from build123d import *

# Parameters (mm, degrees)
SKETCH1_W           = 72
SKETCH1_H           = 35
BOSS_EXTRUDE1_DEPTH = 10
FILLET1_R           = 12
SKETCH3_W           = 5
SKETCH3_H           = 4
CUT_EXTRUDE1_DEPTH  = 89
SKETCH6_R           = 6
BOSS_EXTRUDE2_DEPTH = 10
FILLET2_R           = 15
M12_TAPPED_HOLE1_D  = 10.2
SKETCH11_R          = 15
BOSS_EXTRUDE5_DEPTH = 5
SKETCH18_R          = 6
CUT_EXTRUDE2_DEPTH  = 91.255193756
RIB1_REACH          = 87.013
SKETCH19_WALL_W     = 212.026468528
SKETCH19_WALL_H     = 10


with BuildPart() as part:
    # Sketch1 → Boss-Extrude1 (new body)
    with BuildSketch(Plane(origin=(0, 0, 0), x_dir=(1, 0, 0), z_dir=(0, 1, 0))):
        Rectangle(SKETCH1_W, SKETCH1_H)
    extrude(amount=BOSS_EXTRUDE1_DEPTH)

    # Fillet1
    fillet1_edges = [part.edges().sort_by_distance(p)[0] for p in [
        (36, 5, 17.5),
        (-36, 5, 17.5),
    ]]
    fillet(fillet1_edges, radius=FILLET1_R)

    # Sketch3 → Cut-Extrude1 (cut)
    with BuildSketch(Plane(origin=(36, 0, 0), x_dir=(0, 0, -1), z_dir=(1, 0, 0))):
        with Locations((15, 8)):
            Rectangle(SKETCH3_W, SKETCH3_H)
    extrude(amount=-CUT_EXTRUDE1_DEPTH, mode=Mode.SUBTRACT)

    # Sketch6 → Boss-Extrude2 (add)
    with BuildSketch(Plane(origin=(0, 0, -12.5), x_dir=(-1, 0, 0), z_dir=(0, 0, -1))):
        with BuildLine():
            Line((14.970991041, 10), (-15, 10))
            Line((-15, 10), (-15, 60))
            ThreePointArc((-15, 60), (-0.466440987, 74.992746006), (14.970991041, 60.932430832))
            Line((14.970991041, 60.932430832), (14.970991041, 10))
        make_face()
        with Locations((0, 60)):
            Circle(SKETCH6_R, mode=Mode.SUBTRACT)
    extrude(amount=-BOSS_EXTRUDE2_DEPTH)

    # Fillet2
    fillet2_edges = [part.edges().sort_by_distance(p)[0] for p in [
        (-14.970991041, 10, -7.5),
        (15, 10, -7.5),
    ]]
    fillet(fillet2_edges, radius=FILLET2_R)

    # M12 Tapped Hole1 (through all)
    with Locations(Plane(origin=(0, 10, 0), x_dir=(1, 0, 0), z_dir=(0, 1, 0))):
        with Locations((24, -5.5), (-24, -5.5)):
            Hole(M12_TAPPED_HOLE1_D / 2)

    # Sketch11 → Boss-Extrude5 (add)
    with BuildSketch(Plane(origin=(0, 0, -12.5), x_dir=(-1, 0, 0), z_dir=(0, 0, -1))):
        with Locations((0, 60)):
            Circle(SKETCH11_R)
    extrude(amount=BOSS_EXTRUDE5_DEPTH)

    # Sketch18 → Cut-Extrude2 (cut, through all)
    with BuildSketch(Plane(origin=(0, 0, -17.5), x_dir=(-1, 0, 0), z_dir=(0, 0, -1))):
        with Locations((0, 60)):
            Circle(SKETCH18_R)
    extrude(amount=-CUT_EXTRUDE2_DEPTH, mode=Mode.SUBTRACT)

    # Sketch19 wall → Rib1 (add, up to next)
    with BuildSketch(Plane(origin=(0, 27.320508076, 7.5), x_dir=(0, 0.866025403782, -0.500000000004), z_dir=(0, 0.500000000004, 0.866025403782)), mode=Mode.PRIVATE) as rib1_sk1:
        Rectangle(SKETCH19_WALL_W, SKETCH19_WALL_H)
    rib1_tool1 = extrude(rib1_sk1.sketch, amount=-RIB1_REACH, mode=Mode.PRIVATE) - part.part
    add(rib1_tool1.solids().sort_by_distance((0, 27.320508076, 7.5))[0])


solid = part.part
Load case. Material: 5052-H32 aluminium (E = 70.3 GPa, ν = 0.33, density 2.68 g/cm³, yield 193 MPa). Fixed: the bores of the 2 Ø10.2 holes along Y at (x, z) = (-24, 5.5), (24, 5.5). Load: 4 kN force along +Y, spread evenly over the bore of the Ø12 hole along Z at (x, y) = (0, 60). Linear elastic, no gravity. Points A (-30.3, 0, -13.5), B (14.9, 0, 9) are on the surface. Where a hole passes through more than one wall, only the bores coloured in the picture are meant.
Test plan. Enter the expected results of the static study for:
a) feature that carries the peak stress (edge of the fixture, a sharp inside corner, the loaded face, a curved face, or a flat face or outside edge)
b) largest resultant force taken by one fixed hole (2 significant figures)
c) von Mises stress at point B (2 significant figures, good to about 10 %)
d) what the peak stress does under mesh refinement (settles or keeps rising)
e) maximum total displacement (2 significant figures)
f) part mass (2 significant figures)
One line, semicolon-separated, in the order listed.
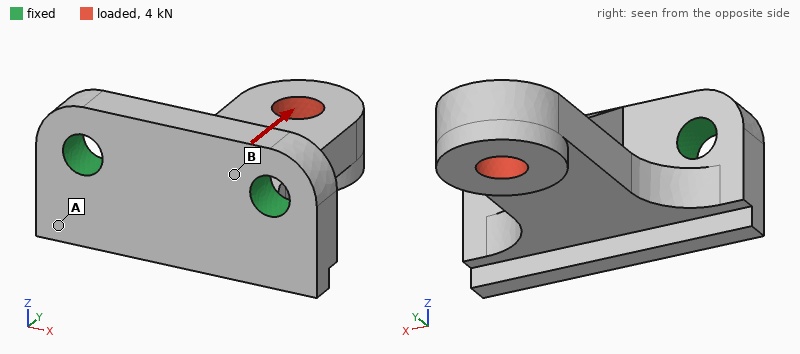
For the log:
edge of the fixture; 2.1 kN; 21 MPa; keeps rising; 0.14 mm; 120 g
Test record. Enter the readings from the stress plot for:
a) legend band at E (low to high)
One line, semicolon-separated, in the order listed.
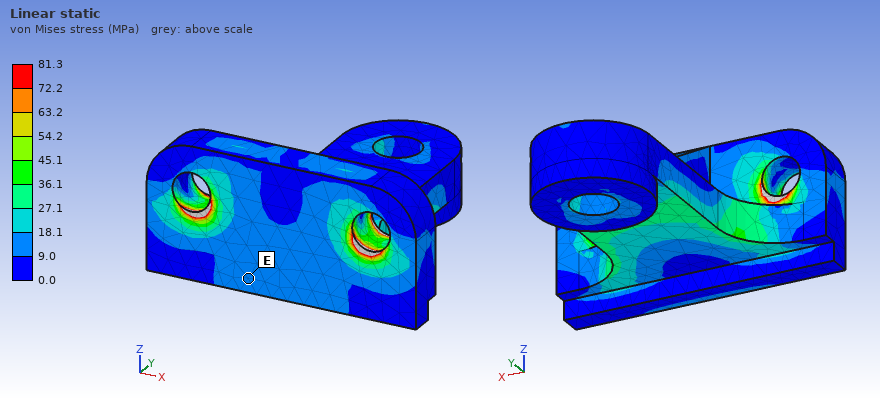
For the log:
9.0 to 18.1 MPa
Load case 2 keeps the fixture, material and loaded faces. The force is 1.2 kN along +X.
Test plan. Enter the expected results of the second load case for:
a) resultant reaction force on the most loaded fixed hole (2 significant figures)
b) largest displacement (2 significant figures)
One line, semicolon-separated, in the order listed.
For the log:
1.7 kN; 67 µm
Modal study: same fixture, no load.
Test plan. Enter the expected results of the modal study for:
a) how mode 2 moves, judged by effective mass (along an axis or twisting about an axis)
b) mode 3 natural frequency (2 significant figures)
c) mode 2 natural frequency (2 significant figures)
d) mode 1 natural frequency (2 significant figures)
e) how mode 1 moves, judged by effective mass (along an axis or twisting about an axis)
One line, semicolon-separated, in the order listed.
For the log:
along X; 8200 Hz; 4500 Hz; 2400 Hz; along Z
